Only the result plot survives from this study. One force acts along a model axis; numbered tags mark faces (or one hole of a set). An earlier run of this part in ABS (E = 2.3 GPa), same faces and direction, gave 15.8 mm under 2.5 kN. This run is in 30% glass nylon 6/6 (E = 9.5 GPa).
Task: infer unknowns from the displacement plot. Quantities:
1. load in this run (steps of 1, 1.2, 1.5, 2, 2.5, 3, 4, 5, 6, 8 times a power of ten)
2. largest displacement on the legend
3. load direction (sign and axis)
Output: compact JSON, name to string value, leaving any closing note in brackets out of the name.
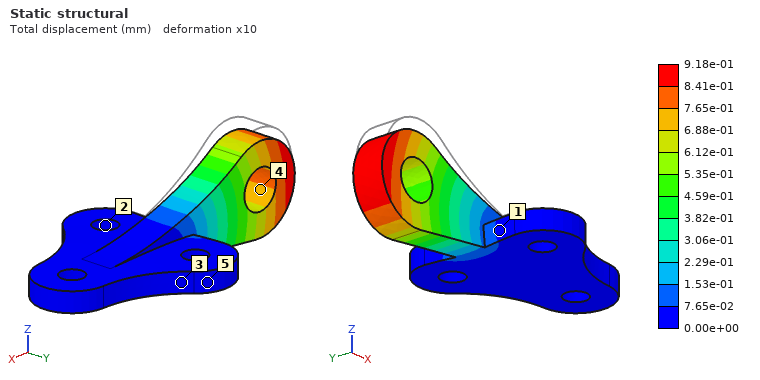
{"load in this run": "600 N", "largest displacement on the legend": "9.18e-01 mm", "load direction": "-Z"}
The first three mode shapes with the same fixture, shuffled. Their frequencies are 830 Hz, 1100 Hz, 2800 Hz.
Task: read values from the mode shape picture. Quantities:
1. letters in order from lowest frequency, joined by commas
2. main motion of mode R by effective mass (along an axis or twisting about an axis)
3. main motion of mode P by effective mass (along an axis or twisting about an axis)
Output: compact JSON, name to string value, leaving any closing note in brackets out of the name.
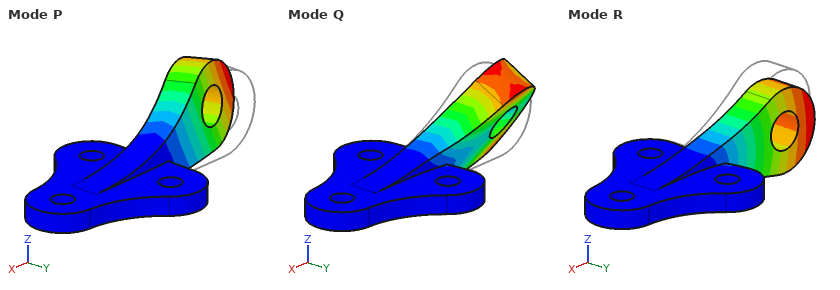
{"letters in order from lowest frequency, joined by commas": "R, P, Q", "main motion of mode R by effective mass": "along Z", "main motion of mode P by effective mass": "along Y"}
